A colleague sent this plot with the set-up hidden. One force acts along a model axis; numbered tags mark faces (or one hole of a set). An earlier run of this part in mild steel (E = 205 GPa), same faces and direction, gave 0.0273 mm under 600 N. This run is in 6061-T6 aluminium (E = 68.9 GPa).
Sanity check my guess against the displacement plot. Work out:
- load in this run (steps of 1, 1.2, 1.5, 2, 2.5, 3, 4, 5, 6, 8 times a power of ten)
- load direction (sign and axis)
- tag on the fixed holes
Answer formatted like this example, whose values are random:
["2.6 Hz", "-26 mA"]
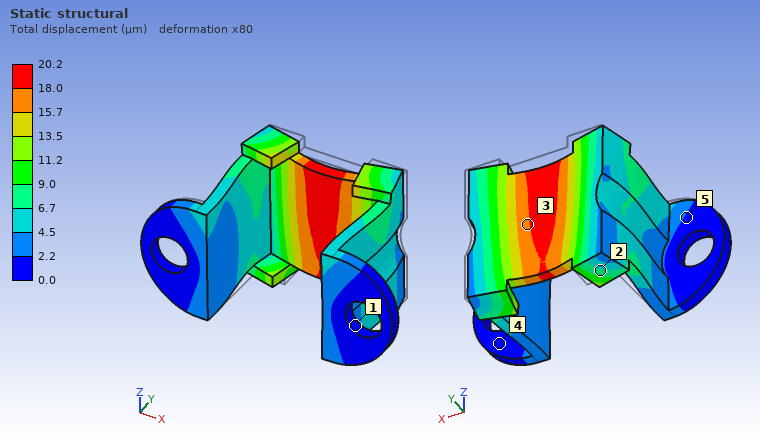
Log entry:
["150 N", "-Y", "1"]
